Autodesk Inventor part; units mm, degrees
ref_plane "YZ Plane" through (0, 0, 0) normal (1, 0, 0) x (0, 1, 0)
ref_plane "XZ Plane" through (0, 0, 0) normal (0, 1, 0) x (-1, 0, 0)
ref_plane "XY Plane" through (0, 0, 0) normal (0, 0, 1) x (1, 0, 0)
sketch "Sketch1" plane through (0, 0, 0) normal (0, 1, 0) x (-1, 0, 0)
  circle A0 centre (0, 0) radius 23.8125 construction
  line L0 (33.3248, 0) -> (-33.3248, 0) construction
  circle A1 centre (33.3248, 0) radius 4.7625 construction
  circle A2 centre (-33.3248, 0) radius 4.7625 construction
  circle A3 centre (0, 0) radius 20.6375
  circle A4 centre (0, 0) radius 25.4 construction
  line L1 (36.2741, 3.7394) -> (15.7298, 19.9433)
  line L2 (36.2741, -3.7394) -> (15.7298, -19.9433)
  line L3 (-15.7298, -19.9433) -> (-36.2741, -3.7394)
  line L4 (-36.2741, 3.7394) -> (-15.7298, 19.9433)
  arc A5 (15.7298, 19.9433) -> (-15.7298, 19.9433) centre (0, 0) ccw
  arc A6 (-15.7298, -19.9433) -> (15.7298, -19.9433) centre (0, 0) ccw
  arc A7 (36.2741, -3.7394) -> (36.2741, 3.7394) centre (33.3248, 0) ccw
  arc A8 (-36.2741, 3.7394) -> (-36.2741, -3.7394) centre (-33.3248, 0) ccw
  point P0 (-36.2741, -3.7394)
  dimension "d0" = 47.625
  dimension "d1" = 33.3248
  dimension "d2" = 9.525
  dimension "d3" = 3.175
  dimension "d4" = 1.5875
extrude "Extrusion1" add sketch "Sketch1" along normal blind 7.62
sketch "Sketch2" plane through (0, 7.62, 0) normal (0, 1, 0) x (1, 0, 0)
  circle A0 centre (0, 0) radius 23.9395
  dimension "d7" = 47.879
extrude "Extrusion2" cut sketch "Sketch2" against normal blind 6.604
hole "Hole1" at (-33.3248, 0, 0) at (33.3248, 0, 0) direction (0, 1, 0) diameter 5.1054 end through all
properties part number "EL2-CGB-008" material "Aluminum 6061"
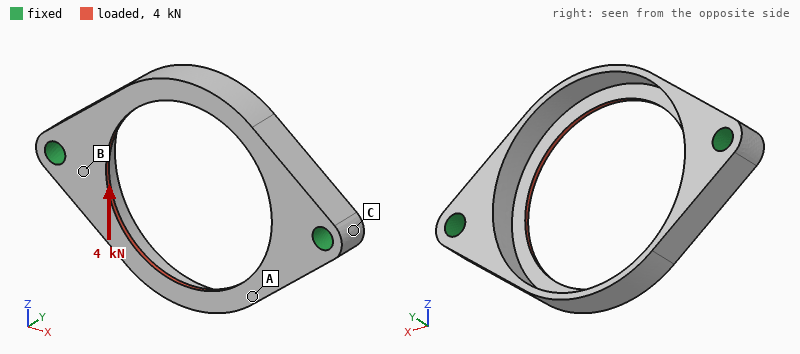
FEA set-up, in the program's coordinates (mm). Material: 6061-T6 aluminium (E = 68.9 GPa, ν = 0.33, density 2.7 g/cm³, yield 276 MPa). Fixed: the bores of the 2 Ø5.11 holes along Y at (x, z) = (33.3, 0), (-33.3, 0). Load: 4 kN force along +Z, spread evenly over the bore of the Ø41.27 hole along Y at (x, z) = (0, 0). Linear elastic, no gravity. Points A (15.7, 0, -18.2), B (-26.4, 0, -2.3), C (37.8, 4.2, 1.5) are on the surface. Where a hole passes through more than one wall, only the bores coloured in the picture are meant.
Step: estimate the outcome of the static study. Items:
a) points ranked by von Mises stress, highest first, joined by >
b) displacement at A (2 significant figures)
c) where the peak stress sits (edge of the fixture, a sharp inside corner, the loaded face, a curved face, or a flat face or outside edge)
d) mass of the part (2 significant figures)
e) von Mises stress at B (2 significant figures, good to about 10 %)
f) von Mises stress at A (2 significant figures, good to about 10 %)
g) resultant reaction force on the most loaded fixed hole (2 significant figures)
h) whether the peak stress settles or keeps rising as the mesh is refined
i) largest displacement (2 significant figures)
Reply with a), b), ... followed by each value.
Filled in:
a) A > B > C
b) 0.068 mm
c) edge of the fixture
d) 14 g
e) 65 MPa
f) 120 MPa
g) 2.0 kN
h) keeps rising
i) 0.14 mm
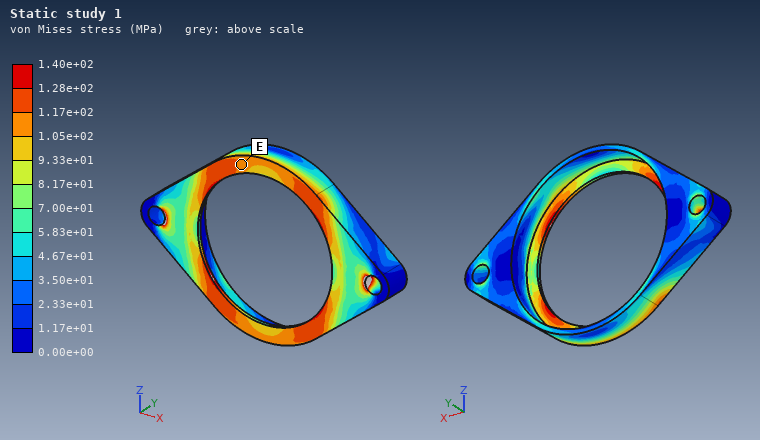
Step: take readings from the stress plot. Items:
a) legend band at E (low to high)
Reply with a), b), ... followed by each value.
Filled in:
a) 1.05e+02 to 1.17e+02 MPa
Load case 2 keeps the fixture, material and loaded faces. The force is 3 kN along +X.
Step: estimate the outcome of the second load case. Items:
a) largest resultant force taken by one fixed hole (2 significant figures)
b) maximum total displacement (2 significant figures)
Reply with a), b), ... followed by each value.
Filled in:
a) 1.5 kN
b) 77 µm
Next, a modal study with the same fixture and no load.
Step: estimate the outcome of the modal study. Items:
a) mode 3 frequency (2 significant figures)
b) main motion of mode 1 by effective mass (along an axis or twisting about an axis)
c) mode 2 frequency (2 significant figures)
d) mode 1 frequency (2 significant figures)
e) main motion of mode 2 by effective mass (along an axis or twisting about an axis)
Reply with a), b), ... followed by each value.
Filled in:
a) 10 kHz
b) twisting about X
c) 7700 Hz
d) 7200 Hz
e) along Y
